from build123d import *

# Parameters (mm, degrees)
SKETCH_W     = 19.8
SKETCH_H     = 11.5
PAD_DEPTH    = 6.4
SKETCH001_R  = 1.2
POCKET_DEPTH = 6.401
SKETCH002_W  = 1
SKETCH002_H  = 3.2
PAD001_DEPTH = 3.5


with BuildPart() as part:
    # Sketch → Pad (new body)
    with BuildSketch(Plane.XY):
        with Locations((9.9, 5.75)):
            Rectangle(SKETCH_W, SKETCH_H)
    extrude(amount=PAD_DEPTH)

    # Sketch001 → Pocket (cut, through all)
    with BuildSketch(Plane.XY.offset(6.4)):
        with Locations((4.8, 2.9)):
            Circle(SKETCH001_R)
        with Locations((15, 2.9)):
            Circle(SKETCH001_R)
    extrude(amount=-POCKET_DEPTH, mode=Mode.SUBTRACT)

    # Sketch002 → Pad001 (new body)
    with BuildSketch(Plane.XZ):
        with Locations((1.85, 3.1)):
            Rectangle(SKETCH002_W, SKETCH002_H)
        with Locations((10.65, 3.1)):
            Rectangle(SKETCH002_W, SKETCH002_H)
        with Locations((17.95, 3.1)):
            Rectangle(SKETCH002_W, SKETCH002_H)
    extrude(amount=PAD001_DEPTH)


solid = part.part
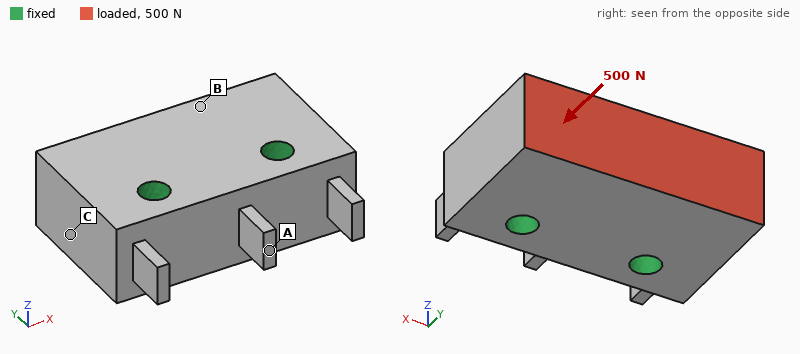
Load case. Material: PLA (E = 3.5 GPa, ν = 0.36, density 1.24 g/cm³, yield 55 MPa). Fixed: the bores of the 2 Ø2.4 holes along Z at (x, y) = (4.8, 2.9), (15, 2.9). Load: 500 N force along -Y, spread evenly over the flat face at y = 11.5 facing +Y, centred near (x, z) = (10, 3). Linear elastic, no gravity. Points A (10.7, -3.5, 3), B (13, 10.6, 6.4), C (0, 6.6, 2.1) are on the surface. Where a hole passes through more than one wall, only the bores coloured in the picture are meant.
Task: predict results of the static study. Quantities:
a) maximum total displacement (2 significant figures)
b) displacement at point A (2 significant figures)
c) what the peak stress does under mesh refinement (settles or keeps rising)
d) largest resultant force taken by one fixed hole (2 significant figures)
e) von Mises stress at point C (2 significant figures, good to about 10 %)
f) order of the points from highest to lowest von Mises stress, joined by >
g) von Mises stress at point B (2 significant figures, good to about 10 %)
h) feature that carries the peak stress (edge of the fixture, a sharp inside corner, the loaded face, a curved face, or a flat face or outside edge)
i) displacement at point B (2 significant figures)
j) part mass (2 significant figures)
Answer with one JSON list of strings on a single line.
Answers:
["15 µm", "3.9 µm", "keeps rising", "250 N", "2.4 MPa", "B > C > A", "4.3 MPa", "edge of the fixture", "10.0 µm", "1.8 g"]
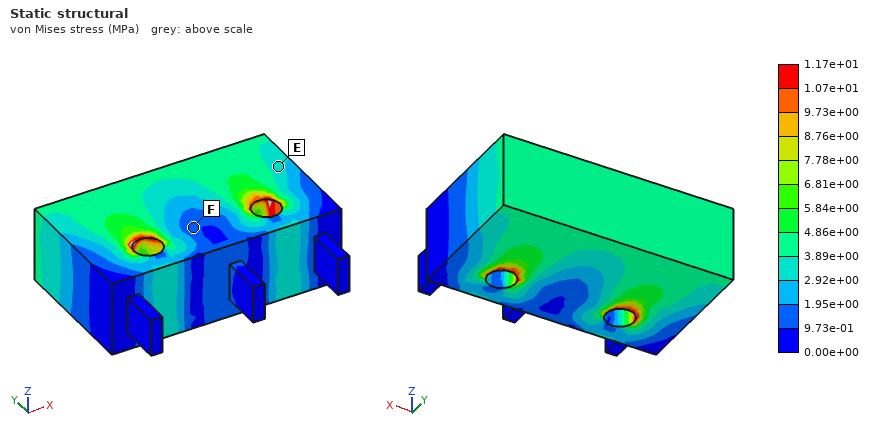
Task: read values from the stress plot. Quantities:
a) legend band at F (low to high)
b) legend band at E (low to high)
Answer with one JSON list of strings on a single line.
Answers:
["9.73e-01 to 1.95e+00 MPa", "2.92e+00 to 3.89e+00 MPa"]
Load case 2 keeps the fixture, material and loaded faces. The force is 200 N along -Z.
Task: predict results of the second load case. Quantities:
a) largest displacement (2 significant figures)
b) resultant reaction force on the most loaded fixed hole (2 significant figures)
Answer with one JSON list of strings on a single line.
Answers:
["51 µm", "100 N"]
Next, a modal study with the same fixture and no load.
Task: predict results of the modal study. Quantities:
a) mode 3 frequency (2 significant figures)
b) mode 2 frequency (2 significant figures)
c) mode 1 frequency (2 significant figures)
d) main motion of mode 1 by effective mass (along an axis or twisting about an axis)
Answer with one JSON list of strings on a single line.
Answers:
["19 kHz", "18 kHz", "16 kHz", "along Z"]
